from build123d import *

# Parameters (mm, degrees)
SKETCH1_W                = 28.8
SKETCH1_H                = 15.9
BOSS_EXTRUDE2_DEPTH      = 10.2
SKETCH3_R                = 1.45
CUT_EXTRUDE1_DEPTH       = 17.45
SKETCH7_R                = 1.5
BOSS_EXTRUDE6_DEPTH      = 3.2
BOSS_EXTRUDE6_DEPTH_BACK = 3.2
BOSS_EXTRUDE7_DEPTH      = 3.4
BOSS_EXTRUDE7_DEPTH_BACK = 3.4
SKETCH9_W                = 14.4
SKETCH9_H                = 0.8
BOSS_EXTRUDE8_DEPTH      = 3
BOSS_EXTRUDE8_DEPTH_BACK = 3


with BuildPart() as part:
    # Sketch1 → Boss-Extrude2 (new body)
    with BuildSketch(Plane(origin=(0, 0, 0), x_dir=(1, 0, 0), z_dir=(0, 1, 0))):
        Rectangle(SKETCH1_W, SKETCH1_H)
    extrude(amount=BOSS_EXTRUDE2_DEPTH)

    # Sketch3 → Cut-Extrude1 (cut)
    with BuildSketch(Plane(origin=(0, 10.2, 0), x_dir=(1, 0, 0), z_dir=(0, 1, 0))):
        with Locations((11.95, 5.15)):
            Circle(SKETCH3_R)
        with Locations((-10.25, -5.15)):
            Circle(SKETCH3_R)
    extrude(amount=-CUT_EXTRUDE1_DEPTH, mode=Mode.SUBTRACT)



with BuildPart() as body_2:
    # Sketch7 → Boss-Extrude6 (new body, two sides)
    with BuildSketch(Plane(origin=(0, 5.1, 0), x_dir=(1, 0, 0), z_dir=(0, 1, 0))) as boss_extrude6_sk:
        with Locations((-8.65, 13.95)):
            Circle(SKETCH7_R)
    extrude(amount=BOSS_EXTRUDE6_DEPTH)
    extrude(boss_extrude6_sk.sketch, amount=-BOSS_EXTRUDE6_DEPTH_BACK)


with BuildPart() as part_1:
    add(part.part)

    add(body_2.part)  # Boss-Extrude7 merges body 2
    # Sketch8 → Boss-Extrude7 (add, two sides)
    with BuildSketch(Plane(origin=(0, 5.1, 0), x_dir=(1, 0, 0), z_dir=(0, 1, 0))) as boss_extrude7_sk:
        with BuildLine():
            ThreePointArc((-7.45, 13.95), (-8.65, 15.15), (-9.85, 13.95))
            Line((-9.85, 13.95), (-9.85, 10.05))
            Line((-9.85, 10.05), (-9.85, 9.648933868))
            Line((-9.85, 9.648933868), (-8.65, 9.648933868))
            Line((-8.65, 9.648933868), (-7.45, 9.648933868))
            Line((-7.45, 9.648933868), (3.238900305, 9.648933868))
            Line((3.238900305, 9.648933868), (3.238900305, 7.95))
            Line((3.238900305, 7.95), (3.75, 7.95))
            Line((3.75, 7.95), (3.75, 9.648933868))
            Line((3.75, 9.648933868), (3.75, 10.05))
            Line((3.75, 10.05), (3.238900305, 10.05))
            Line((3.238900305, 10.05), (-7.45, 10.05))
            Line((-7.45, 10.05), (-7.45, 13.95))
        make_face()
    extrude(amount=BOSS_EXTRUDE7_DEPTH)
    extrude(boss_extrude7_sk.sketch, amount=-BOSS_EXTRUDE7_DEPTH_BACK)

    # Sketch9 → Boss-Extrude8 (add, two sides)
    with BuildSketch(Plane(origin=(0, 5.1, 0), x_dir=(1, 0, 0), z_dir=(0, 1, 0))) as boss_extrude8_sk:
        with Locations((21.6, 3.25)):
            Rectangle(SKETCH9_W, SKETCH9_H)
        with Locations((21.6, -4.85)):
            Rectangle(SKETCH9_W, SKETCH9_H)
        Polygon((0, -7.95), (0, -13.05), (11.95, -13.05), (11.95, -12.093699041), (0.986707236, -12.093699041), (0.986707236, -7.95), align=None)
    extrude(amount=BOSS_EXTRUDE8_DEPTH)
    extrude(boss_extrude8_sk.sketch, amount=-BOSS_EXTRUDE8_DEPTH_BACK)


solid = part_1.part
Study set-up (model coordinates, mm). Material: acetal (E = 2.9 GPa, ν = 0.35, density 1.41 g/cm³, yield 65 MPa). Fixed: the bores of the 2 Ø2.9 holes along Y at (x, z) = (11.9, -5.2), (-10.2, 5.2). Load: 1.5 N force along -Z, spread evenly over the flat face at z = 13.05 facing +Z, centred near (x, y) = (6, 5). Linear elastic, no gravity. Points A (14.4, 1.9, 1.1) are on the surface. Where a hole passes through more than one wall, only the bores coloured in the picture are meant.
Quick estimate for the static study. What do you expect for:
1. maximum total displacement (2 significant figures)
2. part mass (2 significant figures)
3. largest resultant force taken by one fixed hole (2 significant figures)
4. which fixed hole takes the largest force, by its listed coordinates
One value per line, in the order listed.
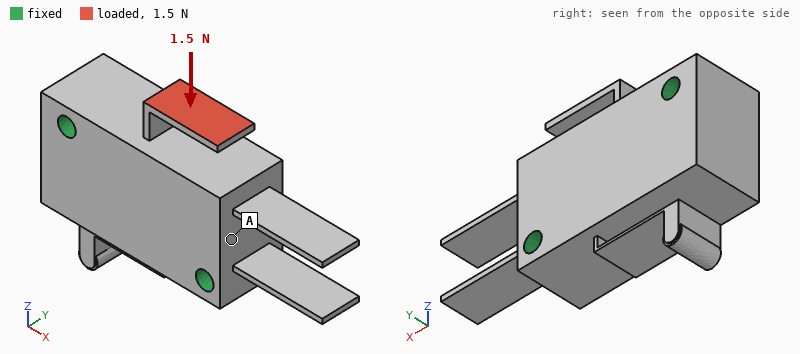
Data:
0.48 mm
6.9 g
1.2 N
(11.9, -5.2)
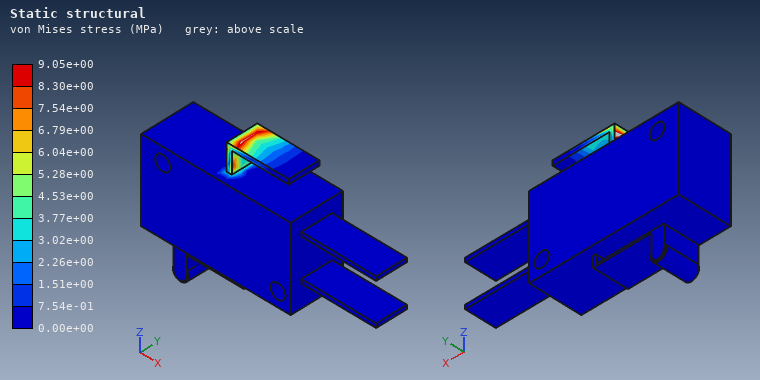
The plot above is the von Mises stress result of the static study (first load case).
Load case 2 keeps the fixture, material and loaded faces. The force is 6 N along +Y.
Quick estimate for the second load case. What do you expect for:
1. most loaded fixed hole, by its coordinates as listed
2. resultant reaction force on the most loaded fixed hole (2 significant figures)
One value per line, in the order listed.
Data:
(-10.2, 5.2)
3.3 N
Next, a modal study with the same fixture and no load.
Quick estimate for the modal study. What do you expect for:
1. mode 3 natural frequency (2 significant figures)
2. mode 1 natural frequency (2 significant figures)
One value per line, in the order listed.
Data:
890 Hz
160 Hz
